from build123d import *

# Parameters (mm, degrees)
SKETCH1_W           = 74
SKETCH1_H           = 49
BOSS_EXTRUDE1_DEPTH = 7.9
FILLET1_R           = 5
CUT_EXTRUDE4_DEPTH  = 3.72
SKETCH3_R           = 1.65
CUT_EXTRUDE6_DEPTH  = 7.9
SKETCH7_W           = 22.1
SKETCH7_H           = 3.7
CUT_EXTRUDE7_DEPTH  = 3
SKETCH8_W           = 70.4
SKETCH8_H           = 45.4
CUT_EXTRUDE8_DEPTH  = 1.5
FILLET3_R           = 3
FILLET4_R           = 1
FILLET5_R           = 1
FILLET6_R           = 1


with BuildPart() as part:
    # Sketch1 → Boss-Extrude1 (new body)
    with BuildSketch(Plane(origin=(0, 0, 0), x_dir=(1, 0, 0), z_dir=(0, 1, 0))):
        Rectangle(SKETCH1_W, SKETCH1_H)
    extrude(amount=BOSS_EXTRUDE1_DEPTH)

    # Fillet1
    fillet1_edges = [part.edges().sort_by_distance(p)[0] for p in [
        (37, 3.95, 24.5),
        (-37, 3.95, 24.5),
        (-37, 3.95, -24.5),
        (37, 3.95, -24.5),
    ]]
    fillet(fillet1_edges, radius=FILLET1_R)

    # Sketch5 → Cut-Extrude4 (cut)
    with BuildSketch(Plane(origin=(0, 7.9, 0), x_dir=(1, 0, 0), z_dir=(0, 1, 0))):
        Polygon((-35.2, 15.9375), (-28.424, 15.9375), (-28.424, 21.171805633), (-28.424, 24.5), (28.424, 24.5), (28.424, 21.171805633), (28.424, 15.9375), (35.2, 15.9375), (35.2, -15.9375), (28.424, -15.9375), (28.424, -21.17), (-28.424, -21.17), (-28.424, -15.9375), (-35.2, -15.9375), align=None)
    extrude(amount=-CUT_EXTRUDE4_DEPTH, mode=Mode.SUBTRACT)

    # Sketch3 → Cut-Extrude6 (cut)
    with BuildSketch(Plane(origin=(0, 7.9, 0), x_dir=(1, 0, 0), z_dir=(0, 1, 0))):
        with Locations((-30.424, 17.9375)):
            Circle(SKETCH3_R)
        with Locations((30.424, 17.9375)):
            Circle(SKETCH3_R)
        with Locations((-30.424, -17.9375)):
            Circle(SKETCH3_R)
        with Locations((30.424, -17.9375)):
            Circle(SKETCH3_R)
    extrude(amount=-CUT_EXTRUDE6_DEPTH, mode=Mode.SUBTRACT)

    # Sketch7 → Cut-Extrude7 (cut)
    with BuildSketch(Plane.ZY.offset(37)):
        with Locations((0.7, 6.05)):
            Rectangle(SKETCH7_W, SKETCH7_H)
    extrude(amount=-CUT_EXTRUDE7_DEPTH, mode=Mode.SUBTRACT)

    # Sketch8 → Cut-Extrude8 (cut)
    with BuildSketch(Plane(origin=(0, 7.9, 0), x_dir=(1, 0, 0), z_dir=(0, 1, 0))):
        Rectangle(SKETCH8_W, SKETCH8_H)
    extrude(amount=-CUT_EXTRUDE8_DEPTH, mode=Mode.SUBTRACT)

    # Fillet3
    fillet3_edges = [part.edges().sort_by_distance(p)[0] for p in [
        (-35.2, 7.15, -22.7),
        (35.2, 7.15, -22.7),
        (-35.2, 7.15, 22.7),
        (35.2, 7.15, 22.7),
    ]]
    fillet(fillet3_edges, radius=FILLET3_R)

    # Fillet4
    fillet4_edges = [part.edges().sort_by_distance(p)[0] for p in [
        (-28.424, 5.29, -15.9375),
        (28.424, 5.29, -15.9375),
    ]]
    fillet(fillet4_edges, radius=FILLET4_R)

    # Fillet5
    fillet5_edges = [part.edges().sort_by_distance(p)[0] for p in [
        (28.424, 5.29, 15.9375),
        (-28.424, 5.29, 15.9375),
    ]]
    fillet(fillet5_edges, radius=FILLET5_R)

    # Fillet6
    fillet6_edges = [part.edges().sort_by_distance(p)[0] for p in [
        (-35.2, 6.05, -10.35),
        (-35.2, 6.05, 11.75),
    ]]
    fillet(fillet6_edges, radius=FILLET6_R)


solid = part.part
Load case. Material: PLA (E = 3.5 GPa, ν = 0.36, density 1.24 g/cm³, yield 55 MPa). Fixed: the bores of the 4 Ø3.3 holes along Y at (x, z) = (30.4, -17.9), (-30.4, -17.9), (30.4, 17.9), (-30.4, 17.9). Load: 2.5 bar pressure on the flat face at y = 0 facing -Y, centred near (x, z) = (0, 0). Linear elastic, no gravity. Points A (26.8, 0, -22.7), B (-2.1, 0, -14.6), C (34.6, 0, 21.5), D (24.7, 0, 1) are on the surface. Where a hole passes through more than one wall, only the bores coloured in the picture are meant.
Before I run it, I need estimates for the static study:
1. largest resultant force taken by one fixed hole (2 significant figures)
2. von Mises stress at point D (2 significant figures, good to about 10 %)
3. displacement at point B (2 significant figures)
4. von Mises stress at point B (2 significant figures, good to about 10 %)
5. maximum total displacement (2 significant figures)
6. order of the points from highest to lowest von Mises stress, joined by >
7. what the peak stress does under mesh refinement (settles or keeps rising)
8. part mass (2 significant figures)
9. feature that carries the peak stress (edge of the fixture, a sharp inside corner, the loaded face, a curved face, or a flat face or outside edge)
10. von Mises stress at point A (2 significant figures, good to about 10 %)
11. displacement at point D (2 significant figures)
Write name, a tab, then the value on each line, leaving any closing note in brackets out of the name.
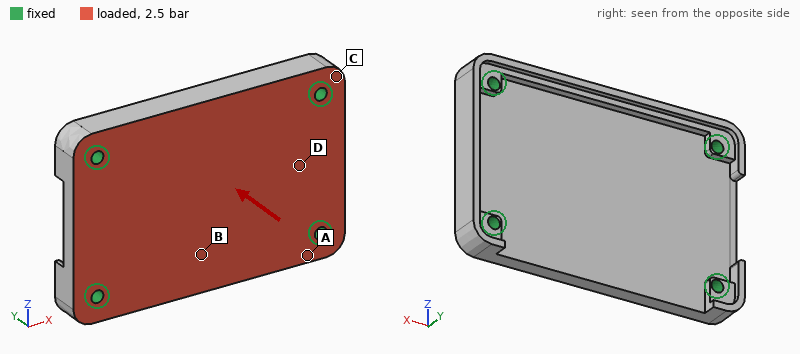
largest resultant force taken by one fixed hole	230 N
von Mises stress at point D	6.2 MPa
displacement at point B	0.49 mm
von Mises stress at point B	13 MPa
maximum total displacement	0.51 mm
order of the points from highest to lowest von Mises stress, joined by >	A > B > D > C
what the peak stress does under mesh refinement	keeps rising
part mass	20 g
feature that carries the peak stress	edge of the fixture
von Mises stress at point A	18 MPa
displacement at point D	0.16 mm
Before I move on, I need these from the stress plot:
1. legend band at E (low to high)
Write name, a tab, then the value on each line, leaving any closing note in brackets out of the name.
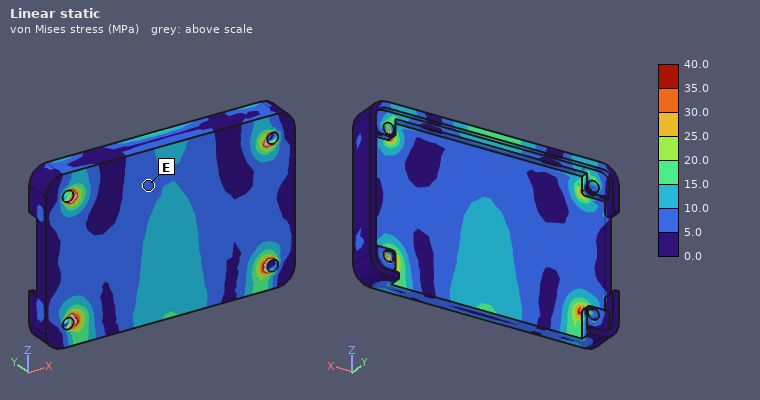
legend band at E	5.0 to 10.0 MPa
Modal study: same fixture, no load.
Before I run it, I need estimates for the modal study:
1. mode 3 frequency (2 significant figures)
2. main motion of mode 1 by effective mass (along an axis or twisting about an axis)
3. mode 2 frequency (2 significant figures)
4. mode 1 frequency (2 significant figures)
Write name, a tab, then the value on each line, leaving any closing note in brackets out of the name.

mode 3 frequency	4200 Hz
main motion of mode 1 by effective mass	along Y
mode 2 frequency	2700 Hz
mode 1 frequency	1800 Hz
